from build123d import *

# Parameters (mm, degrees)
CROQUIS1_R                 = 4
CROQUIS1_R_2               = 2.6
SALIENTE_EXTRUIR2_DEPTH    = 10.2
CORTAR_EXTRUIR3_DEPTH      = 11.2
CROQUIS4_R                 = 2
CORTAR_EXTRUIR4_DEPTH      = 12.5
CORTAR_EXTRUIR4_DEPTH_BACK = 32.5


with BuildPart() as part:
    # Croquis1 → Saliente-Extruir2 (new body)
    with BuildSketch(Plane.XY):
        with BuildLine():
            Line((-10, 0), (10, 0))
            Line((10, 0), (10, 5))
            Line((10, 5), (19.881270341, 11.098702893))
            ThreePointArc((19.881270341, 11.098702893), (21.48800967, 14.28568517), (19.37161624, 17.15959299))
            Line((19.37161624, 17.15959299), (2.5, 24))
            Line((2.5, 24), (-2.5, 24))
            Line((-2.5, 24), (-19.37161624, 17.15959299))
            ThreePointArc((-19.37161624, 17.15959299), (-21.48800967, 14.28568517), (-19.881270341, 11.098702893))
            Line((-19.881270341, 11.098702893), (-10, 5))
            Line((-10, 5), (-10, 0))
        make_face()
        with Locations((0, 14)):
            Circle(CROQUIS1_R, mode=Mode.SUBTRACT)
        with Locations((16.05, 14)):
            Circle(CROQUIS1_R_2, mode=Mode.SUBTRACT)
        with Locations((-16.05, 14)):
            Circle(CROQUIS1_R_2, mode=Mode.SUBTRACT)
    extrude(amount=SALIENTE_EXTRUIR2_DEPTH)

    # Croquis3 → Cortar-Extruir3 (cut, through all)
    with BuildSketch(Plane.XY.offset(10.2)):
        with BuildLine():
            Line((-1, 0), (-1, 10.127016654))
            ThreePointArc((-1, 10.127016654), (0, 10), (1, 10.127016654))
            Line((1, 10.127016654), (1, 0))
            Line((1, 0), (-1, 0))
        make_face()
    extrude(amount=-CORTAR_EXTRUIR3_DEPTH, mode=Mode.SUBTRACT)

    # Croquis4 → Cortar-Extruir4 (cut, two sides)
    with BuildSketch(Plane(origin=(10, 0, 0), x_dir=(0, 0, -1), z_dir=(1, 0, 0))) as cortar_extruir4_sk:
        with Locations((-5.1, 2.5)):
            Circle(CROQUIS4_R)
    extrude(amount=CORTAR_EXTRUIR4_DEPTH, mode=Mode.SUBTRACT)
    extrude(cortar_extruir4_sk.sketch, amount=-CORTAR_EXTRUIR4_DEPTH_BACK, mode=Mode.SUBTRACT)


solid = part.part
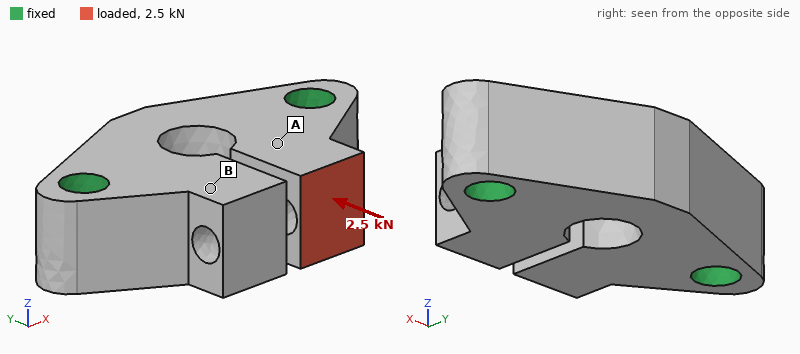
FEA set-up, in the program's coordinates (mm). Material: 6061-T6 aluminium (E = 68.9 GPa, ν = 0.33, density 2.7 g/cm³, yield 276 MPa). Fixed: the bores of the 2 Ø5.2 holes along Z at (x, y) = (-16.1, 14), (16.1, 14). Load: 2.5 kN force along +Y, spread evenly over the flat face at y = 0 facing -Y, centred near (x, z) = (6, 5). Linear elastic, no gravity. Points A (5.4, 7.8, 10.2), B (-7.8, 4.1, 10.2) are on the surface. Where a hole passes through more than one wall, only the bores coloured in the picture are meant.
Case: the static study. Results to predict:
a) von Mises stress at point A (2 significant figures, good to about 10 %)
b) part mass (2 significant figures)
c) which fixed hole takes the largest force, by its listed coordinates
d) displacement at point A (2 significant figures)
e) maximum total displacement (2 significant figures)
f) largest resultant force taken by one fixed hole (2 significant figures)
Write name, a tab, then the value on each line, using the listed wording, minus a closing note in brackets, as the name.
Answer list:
von Mises stress at point A	50 MPa
part mass	15 g
which fixed hole takes the largest force, by its listed coordinates	(16.1, 14)
displacement at point A	17 µm
maximum total displacement	43 µm
largest resultant force taken by one fixed hole	2.1 kN
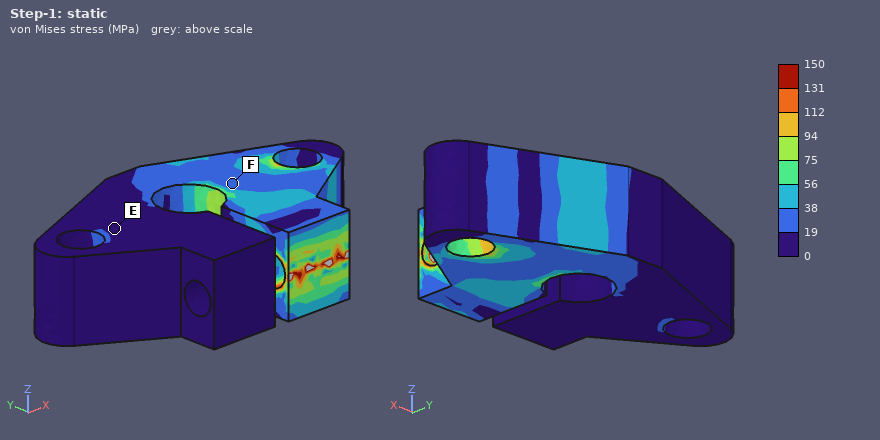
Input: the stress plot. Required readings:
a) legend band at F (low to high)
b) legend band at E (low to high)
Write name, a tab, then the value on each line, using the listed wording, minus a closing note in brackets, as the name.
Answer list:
legend band at F	19 to 38 MPa
legend band at E	0 to 19 MPa
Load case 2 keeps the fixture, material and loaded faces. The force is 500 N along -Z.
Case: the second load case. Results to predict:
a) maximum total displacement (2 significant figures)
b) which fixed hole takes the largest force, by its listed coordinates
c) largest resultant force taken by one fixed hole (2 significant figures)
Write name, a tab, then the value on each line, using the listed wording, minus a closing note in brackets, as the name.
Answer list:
maximum total displacement	24 µm
which fixed hole takes the largest force, by its listed coordinates	(16.1, 14)
largest resultant force taken by one fixed hole	500 N
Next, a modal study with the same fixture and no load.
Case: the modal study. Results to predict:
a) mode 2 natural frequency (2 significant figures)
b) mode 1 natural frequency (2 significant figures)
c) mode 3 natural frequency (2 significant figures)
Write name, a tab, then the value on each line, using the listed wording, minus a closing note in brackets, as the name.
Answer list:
mode 2 natural frequency	24 kHz
mode 1 natural frequency	24 kHz
mode 3 natural frequency	25 kHz
